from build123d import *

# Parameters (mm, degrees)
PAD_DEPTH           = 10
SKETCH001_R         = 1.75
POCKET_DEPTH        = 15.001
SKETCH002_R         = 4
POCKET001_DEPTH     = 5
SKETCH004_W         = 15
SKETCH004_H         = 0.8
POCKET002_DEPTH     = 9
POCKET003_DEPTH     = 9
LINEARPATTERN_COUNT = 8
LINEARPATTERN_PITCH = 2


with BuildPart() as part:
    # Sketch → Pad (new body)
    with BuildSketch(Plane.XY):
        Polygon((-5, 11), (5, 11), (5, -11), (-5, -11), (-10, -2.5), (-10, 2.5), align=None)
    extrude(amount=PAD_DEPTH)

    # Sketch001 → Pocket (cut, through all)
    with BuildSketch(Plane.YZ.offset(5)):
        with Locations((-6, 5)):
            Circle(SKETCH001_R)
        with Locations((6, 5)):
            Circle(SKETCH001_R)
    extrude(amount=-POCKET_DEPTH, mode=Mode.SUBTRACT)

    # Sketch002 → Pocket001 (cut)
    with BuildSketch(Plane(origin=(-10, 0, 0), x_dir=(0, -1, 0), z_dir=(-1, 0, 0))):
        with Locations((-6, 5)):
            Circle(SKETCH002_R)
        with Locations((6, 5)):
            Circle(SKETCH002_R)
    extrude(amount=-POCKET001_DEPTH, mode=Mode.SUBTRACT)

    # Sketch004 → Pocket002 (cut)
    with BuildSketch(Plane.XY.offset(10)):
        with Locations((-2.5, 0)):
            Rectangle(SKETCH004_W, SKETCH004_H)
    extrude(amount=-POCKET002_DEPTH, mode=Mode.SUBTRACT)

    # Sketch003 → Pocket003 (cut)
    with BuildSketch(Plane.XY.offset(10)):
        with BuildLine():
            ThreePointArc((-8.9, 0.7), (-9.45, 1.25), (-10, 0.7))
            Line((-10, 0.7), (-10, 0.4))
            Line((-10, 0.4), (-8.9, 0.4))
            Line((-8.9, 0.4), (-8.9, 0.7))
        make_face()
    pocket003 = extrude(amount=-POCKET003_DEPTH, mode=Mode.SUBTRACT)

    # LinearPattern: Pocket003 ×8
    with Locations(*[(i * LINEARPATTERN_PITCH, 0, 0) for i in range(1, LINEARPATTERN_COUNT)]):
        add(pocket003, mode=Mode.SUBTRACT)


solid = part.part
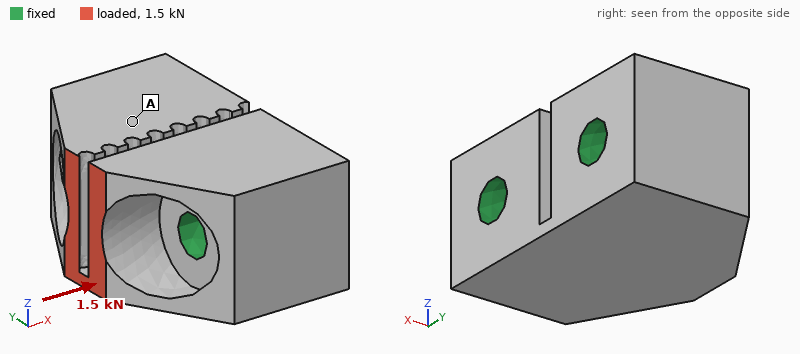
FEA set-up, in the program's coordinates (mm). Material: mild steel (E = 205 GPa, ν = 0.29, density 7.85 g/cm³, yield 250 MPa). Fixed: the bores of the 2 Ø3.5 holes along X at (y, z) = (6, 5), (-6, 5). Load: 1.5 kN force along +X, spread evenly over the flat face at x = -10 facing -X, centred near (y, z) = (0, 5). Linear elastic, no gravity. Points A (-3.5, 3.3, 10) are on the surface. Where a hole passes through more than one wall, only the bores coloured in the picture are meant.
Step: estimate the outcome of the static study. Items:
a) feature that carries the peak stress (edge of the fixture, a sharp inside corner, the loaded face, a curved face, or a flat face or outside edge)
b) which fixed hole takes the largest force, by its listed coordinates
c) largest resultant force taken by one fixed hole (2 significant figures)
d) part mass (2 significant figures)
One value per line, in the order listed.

the loaded face
(-6, 5)
800 N
17 g
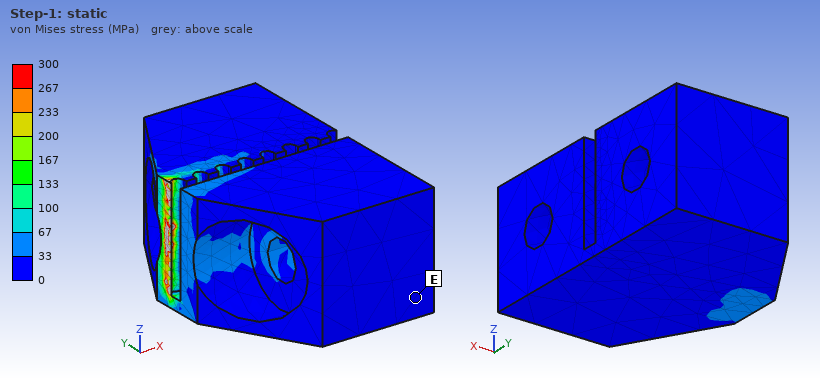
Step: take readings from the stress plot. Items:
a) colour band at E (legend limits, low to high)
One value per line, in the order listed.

0 to 33 MPa
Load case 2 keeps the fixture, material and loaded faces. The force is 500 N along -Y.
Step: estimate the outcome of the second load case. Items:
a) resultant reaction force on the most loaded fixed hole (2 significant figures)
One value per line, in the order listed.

290 N
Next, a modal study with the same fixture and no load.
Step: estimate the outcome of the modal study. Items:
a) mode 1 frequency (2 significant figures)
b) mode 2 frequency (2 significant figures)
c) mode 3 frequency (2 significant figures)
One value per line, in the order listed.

62 kHz
67 kHz
71 kHz
